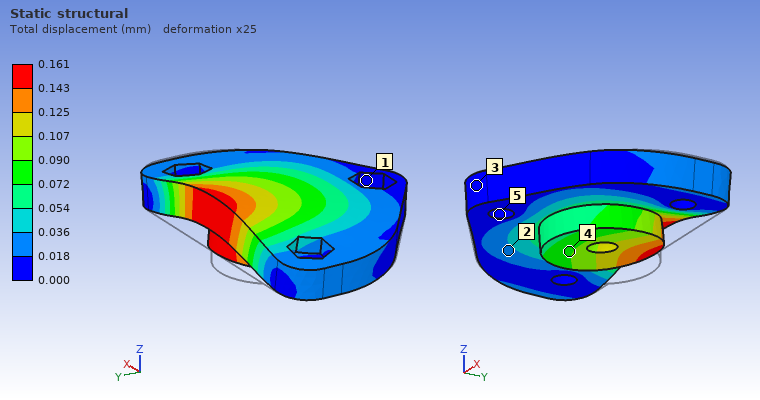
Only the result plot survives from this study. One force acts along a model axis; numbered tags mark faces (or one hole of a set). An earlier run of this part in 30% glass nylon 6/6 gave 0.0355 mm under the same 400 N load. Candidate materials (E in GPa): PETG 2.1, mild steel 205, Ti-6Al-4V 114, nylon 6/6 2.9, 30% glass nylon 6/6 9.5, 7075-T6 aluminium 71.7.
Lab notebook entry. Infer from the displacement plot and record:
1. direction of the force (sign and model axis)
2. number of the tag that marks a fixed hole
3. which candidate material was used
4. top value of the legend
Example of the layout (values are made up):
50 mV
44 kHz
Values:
+Z
5
PETG
0.161 mm
